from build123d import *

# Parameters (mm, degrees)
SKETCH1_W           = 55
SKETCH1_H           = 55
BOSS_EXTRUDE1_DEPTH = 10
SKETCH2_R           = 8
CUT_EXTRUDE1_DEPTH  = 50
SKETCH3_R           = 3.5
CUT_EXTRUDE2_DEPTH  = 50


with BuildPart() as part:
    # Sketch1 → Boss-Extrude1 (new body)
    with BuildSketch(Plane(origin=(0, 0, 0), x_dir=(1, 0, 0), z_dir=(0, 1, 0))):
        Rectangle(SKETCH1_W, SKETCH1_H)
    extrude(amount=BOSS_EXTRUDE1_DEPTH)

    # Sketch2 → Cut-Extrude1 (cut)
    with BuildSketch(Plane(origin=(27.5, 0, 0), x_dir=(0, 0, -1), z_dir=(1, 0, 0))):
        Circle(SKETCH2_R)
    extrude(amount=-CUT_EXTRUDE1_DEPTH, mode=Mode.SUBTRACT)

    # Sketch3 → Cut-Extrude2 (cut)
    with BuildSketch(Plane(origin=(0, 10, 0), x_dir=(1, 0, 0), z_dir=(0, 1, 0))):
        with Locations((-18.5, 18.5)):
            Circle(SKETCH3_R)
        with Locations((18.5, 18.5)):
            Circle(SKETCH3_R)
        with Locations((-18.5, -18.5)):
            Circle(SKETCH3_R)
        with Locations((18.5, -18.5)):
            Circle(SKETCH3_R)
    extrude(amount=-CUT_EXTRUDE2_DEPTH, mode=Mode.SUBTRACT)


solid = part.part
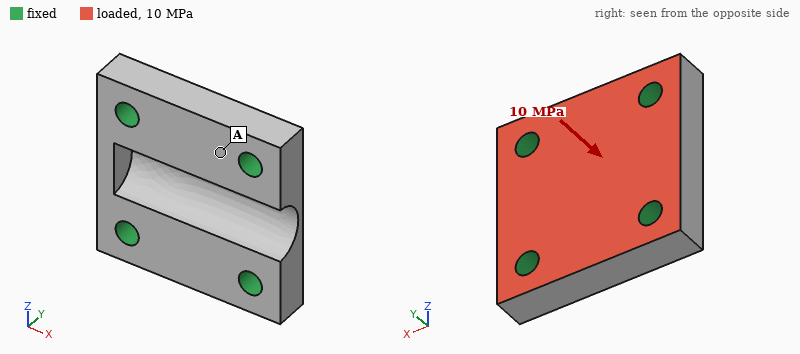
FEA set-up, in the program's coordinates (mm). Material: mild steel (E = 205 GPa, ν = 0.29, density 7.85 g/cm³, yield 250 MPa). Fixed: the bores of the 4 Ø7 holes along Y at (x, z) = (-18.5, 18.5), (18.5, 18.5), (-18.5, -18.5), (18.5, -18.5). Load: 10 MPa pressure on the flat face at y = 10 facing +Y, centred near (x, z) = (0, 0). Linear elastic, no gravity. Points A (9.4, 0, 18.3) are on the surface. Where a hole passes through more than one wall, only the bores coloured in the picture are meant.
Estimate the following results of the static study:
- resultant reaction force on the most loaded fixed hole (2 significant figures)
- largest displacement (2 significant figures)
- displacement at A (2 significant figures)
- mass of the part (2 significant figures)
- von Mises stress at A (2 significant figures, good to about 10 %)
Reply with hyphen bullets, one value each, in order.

- 7.6 kN
- 14 µm
- 3.9 µm
- 190 g
- 31 MPa
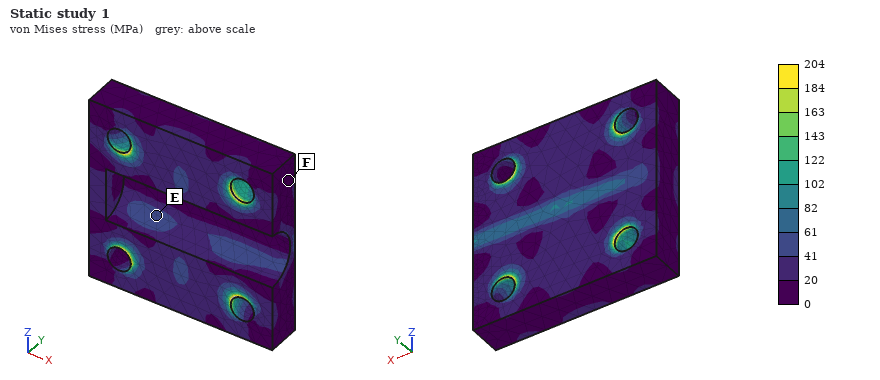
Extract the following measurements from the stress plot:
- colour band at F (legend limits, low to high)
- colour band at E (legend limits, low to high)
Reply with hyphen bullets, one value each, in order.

- 0 to 20 MPa
- 41 to 61 MPa
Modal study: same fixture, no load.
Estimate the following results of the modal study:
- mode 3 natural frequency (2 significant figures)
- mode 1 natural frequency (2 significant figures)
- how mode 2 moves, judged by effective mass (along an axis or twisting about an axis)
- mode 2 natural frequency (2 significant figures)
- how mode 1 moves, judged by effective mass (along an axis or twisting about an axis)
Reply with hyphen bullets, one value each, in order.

- 33 kHz
- 26 kHz
- twisting about X
- 31 kHz
- along Y
